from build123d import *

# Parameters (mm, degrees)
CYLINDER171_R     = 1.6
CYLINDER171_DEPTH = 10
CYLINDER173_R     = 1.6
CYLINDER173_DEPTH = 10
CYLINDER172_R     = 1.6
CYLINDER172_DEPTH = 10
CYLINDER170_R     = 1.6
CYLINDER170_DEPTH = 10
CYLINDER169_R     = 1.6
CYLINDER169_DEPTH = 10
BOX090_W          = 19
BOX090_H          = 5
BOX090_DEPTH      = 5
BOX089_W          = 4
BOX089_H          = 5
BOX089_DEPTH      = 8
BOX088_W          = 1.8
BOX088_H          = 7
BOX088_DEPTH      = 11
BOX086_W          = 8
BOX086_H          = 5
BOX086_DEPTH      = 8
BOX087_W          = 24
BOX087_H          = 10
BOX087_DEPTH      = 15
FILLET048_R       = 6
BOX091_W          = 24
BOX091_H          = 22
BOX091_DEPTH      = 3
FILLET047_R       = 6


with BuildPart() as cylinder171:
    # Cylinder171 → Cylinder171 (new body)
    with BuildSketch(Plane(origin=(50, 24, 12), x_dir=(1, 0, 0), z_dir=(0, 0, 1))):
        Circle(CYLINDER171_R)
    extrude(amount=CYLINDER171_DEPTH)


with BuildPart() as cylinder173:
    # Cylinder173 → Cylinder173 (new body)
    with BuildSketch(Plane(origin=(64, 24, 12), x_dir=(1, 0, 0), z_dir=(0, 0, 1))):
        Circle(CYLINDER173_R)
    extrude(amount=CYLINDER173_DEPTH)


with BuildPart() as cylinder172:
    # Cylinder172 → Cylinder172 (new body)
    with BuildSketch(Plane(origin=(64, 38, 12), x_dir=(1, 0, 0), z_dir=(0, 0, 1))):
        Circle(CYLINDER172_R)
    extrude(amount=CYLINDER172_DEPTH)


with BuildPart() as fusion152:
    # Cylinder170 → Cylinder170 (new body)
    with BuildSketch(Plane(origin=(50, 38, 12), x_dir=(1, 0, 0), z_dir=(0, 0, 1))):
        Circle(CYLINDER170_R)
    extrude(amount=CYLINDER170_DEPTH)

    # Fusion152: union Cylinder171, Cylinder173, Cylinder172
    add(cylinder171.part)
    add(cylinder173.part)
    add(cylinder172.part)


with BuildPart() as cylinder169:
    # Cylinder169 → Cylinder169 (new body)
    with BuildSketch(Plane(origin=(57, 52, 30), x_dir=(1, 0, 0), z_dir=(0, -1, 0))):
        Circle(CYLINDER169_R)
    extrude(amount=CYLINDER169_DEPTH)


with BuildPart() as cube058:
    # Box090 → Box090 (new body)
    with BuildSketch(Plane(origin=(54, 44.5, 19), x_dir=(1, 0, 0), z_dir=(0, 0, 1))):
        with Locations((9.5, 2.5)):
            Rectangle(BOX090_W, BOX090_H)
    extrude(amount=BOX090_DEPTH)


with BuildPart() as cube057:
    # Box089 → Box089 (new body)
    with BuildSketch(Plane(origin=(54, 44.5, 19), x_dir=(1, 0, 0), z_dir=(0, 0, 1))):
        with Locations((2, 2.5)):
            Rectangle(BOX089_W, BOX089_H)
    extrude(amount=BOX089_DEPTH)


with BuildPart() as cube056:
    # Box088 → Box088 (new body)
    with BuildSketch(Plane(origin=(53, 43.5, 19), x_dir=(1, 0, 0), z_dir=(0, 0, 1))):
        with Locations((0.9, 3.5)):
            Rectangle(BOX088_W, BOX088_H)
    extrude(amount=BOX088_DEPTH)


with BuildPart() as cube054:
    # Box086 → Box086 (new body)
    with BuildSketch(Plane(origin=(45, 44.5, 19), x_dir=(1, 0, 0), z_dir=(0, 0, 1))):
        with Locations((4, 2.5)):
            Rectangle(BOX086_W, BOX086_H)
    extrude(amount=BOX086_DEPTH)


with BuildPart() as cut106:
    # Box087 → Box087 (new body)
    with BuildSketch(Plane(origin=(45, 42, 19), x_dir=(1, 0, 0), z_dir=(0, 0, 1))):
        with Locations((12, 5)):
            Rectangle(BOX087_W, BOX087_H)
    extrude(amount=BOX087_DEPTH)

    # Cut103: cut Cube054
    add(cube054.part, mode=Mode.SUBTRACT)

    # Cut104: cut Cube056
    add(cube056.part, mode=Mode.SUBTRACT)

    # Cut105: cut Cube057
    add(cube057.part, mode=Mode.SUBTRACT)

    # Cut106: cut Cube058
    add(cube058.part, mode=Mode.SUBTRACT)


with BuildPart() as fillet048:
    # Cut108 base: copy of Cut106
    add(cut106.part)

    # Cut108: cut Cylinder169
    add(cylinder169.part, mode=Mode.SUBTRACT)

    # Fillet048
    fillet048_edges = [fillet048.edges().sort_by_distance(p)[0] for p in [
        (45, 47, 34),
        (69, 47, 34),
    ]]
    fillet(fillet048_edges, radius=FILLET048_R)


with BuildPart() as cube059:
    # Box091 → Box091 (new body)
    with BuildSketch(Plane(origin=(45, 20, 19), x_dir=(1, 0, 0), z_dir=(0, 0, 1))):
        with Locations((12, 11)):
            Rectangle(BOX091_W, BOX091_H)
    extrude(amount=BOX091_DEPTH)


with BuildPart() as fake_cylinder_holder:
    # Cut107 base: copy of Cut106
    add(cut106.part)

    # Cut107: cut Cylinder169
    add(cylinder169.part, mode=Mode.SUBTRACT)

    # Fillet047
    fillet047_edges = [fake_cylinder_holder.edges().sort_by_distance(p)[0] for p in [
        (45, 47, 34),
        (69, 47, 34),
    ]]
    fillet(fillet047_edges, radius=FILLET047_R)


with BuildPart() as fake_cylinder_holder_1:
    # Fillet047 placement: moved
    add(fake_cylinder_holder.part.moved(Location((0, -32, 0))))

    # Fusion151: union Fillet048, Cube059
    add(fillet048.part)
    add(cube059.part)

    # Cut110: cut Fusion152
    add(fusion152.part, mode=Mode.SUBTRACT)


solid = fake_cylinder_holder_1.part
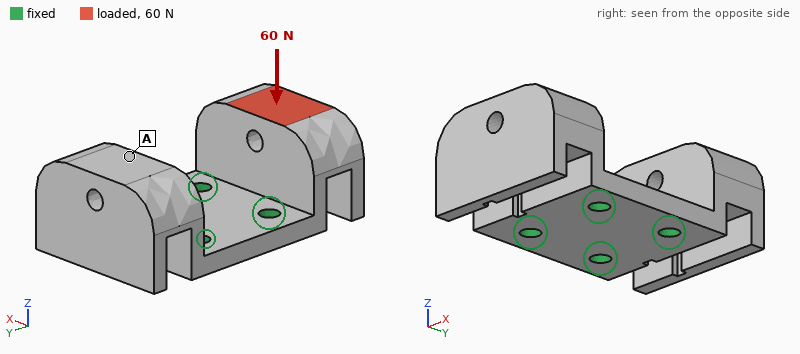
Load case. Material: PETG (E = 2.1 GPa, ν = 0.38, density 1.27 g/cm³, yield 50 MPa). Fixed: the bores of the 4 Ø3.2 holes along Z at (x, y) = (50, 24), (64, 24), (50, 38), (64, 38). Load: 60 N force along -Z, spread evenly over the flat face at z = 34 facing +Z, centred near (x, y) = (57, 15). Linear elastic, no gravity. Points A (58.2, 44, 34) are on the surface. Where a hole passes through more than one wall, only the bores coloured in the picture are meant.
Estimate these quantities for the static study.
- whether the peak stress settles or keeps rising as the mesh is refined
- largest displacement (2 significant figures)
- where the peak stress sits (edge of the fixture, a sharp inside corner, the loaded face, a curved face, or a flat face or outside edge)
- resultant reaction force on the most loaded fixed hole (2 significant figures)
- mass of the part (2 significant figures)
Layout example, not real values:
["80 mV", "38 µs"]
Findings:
["keeps rising", "0.49 mm", "edge of the fixture", "34 N", "8.2 g"]
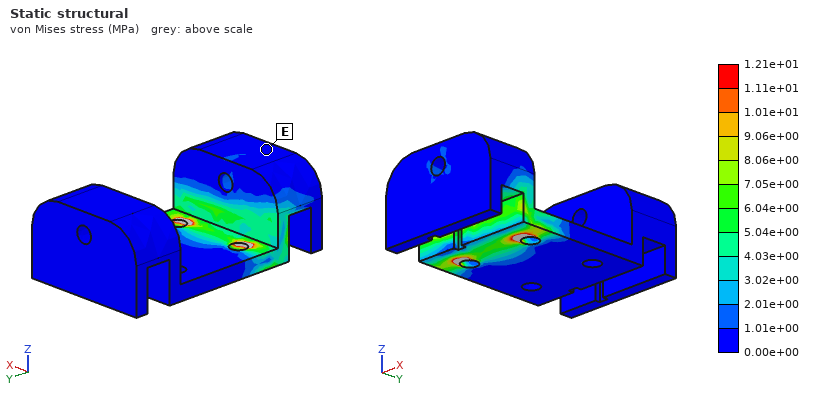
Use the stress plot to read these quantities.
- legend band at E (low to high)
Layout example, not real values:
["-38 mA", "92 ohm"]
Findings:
["0.00e+00 to 1.01e+00 MPa"]
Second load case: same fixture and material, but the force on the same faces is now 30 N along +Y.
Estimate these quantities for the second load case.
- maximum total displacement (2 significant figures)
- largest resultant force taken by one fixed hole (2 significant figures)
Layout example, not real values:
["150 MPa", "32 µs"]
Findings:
["0.58 mm", "15 N"]
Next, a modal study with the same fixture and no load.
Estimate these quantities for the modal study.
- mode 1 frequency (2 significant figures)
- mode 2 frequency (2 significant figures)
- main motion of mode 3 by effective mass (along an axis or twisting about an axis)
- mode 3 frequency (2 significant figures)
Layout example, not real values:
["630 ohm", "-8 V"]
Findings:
["990 Hz", "990 Hz", "twisting about Z", "2900 Hz"]
